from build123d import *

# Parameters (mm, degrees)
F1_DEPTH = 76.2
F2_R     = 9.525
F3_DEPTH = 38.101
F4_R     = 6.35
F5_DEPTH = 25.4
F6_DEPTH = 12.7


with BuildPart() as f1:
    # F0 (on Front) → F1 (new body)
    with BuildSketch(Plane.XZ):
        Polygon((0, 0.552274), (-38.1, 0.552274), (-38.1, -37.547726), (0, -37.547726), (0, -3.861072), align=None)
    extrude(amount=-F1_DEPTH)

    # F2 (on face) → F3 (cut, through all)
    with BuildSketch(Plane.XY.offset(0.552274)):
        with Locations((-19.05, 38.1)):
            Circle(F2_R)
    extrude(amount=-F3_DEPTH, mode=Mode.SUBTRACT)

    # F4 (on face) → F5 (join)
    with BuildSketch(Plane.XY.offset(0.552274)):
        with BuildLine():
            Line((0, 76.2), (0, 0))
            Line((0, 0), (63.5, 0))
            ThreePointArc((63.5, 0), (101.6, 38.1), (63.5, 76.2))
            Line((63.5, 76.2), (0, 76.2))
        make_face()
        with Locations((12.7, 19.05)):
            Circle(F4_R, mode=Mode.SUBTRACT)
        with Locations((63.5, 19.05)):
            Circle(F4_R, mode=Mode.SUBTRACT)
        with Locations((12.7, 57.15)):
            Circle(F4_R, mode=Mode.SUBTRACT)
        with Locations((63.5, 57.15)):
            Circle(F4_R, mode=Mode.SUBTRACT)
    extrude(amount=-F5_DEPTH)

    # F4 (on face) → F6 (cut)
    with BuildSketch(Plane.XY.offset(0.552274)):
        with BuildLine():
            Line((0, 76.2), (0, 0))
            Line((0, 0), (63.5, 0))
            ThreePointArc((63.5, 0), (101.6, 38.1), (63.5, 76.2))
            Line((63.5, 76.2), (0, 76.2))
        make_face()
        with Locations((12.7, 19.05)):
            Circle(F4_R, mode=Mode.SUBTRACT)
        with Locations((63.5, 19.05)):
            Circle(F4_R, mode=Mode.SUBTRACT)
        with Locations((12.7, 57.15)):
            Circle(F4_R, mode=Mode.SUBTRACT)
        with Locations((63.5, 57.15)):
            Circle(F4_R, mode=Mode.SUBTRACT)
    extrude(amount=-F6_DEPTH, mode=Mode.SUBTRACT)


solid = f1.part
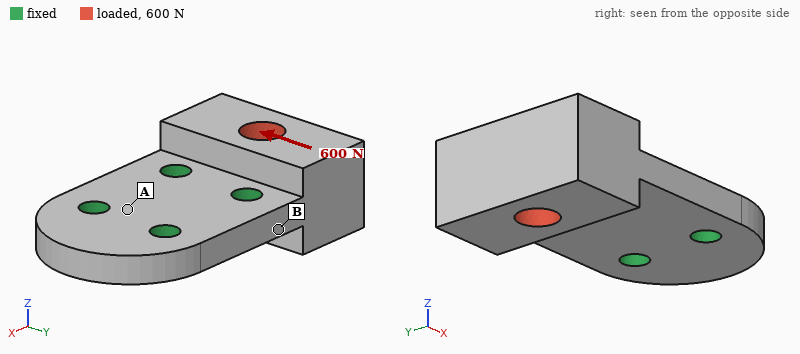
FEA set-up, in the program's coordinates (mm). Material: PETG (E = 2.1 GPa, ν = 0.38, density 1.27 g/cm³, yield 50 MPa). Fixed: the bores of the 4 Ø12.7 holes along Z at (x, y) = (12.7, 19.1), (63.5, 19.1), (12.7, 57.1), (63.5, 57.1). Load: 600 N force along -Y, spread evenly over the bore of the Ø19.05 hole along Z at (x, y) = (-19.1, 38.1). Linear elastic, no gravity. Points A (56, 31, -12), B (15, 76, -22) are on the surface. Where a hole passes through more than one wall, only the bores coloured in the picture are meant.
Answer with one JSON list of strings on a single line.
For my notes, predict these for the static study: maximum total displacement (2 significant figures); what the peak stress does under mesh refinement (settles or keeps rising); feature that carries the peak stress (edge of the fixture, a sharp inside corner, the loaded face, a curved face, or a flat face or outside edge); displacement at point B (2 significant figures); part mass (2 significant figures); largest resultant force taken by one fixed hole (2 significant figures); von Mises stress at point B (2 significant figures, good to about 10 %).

["45 µm", "keeps rising", "edge of the fixture", "8.2 µm", "230 g", "440 N", "1.1 MPa"]
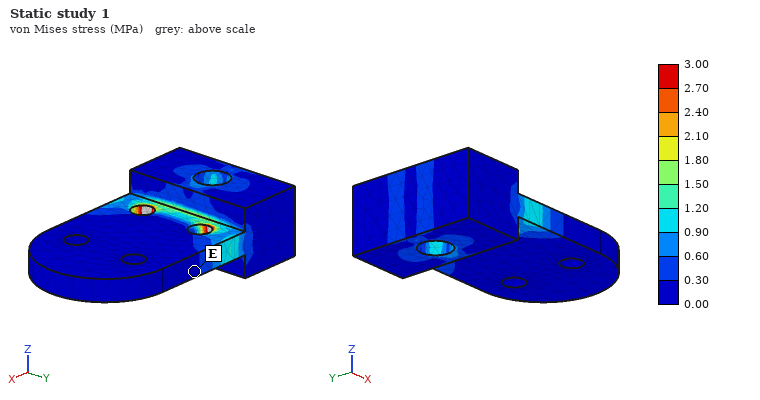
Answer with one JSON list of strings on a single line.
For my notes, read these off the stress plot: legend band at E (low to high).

["0.00 to 0.30 MPa"]
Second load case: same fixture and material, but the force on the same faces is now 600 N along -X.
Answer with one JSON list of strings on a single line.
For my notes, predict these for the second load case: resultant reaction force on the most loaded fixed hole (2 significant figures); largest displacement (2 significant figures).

["290 N", "15 µm"]
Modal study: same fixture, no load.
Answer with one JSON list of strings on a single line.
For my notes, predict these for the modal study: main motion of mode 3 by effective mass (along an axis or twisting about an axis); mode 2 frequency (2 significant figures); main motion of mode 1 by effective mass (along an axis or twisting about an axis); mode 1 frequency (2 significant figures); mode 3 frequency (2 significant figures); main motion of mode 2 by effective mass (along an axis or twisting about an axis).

["along Y", "1600 Hz", "along Z", "700 Hz", "1900 Hz", "twisting about X"]
